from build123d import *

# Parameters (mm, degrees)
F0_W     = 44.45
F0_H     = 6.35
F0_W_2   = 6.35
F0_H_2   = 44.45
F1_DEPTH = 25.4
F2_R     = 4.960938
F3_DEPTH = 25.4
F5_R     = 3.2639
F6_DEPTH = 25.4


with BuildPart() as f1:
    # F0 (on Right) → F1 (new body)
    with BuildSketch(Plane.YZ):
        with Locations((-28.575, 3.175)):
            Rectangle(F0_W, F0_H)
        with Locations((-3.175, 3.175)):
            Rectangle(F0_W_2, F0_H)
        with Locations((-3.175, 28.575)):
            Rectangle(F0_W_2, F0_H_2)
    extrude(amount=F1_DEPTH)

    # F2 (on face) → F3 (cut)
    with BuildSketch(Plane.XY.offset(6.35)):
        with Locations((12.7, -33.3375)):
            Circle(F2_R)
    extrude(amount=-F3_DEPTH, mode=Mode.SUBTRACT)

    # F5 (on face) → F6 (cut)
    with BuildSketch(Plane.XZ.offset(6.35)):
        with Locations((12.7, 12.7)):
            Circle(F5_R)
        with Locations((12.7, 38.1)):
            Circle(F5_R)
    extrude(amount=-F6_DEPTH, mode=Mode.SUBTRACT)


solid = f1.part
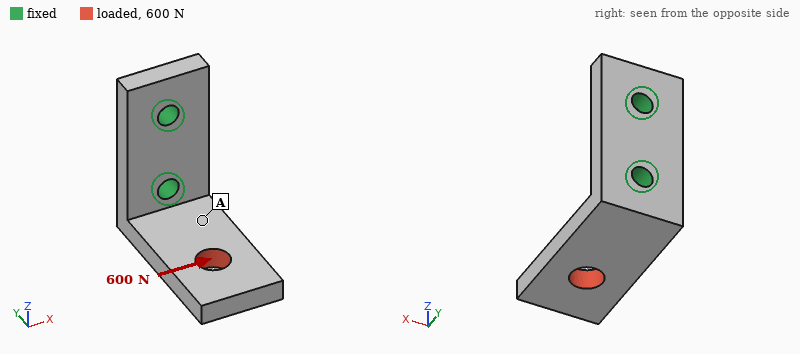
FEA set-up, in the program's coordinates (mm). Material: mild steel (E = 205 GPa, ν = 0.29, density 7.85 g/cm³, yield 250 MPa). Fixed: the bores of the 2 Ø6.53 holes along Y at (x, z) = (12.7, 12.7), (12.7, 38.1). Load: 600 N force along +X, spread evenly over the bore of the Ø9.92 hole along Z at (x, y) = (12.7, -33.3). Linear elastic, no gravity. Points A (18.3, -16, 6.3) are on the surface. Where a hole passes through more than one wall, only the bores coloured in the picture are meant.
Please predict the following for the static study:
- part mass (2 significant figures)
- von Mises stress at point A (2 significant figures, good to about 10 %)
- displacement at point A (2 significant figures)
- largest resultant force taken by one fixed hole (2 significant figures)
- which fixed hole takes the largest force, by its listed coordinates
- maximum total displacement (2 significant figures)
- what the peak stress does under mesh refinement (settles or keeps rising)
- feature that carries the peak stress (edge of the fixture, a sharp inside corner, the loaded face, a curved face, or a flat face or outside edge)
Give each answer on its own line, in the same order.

110 g
17 MPa
12 µm
720 N
(12.7, 12.7)
45 µm
keeps rising
edge of the fixture
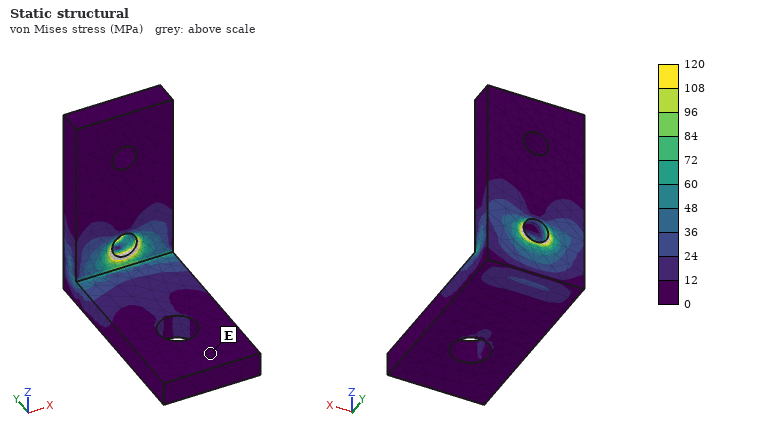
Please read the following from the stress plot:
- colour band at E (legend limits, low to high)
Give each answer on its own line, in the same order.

0 to 12 MPa
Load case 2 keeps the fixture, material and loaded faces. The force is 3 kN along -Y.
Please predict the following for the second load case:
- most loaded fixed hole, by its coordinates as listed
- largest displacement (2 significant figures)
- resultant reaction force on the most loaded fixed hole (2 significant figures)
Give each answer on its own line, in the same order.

(12.7, 12.7)
56 µm
3.2 kN
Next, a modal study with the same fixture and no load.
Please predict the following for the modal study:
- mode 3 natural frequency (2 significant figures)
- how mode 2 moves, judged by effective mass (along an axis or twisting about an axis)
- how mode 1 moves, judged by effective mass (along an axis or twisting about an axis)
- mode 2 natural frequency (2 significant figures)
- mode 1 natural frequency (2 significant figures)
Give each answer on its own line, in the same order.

7600 Hz
along X
along Z
3400 Hz
1900 Hz
